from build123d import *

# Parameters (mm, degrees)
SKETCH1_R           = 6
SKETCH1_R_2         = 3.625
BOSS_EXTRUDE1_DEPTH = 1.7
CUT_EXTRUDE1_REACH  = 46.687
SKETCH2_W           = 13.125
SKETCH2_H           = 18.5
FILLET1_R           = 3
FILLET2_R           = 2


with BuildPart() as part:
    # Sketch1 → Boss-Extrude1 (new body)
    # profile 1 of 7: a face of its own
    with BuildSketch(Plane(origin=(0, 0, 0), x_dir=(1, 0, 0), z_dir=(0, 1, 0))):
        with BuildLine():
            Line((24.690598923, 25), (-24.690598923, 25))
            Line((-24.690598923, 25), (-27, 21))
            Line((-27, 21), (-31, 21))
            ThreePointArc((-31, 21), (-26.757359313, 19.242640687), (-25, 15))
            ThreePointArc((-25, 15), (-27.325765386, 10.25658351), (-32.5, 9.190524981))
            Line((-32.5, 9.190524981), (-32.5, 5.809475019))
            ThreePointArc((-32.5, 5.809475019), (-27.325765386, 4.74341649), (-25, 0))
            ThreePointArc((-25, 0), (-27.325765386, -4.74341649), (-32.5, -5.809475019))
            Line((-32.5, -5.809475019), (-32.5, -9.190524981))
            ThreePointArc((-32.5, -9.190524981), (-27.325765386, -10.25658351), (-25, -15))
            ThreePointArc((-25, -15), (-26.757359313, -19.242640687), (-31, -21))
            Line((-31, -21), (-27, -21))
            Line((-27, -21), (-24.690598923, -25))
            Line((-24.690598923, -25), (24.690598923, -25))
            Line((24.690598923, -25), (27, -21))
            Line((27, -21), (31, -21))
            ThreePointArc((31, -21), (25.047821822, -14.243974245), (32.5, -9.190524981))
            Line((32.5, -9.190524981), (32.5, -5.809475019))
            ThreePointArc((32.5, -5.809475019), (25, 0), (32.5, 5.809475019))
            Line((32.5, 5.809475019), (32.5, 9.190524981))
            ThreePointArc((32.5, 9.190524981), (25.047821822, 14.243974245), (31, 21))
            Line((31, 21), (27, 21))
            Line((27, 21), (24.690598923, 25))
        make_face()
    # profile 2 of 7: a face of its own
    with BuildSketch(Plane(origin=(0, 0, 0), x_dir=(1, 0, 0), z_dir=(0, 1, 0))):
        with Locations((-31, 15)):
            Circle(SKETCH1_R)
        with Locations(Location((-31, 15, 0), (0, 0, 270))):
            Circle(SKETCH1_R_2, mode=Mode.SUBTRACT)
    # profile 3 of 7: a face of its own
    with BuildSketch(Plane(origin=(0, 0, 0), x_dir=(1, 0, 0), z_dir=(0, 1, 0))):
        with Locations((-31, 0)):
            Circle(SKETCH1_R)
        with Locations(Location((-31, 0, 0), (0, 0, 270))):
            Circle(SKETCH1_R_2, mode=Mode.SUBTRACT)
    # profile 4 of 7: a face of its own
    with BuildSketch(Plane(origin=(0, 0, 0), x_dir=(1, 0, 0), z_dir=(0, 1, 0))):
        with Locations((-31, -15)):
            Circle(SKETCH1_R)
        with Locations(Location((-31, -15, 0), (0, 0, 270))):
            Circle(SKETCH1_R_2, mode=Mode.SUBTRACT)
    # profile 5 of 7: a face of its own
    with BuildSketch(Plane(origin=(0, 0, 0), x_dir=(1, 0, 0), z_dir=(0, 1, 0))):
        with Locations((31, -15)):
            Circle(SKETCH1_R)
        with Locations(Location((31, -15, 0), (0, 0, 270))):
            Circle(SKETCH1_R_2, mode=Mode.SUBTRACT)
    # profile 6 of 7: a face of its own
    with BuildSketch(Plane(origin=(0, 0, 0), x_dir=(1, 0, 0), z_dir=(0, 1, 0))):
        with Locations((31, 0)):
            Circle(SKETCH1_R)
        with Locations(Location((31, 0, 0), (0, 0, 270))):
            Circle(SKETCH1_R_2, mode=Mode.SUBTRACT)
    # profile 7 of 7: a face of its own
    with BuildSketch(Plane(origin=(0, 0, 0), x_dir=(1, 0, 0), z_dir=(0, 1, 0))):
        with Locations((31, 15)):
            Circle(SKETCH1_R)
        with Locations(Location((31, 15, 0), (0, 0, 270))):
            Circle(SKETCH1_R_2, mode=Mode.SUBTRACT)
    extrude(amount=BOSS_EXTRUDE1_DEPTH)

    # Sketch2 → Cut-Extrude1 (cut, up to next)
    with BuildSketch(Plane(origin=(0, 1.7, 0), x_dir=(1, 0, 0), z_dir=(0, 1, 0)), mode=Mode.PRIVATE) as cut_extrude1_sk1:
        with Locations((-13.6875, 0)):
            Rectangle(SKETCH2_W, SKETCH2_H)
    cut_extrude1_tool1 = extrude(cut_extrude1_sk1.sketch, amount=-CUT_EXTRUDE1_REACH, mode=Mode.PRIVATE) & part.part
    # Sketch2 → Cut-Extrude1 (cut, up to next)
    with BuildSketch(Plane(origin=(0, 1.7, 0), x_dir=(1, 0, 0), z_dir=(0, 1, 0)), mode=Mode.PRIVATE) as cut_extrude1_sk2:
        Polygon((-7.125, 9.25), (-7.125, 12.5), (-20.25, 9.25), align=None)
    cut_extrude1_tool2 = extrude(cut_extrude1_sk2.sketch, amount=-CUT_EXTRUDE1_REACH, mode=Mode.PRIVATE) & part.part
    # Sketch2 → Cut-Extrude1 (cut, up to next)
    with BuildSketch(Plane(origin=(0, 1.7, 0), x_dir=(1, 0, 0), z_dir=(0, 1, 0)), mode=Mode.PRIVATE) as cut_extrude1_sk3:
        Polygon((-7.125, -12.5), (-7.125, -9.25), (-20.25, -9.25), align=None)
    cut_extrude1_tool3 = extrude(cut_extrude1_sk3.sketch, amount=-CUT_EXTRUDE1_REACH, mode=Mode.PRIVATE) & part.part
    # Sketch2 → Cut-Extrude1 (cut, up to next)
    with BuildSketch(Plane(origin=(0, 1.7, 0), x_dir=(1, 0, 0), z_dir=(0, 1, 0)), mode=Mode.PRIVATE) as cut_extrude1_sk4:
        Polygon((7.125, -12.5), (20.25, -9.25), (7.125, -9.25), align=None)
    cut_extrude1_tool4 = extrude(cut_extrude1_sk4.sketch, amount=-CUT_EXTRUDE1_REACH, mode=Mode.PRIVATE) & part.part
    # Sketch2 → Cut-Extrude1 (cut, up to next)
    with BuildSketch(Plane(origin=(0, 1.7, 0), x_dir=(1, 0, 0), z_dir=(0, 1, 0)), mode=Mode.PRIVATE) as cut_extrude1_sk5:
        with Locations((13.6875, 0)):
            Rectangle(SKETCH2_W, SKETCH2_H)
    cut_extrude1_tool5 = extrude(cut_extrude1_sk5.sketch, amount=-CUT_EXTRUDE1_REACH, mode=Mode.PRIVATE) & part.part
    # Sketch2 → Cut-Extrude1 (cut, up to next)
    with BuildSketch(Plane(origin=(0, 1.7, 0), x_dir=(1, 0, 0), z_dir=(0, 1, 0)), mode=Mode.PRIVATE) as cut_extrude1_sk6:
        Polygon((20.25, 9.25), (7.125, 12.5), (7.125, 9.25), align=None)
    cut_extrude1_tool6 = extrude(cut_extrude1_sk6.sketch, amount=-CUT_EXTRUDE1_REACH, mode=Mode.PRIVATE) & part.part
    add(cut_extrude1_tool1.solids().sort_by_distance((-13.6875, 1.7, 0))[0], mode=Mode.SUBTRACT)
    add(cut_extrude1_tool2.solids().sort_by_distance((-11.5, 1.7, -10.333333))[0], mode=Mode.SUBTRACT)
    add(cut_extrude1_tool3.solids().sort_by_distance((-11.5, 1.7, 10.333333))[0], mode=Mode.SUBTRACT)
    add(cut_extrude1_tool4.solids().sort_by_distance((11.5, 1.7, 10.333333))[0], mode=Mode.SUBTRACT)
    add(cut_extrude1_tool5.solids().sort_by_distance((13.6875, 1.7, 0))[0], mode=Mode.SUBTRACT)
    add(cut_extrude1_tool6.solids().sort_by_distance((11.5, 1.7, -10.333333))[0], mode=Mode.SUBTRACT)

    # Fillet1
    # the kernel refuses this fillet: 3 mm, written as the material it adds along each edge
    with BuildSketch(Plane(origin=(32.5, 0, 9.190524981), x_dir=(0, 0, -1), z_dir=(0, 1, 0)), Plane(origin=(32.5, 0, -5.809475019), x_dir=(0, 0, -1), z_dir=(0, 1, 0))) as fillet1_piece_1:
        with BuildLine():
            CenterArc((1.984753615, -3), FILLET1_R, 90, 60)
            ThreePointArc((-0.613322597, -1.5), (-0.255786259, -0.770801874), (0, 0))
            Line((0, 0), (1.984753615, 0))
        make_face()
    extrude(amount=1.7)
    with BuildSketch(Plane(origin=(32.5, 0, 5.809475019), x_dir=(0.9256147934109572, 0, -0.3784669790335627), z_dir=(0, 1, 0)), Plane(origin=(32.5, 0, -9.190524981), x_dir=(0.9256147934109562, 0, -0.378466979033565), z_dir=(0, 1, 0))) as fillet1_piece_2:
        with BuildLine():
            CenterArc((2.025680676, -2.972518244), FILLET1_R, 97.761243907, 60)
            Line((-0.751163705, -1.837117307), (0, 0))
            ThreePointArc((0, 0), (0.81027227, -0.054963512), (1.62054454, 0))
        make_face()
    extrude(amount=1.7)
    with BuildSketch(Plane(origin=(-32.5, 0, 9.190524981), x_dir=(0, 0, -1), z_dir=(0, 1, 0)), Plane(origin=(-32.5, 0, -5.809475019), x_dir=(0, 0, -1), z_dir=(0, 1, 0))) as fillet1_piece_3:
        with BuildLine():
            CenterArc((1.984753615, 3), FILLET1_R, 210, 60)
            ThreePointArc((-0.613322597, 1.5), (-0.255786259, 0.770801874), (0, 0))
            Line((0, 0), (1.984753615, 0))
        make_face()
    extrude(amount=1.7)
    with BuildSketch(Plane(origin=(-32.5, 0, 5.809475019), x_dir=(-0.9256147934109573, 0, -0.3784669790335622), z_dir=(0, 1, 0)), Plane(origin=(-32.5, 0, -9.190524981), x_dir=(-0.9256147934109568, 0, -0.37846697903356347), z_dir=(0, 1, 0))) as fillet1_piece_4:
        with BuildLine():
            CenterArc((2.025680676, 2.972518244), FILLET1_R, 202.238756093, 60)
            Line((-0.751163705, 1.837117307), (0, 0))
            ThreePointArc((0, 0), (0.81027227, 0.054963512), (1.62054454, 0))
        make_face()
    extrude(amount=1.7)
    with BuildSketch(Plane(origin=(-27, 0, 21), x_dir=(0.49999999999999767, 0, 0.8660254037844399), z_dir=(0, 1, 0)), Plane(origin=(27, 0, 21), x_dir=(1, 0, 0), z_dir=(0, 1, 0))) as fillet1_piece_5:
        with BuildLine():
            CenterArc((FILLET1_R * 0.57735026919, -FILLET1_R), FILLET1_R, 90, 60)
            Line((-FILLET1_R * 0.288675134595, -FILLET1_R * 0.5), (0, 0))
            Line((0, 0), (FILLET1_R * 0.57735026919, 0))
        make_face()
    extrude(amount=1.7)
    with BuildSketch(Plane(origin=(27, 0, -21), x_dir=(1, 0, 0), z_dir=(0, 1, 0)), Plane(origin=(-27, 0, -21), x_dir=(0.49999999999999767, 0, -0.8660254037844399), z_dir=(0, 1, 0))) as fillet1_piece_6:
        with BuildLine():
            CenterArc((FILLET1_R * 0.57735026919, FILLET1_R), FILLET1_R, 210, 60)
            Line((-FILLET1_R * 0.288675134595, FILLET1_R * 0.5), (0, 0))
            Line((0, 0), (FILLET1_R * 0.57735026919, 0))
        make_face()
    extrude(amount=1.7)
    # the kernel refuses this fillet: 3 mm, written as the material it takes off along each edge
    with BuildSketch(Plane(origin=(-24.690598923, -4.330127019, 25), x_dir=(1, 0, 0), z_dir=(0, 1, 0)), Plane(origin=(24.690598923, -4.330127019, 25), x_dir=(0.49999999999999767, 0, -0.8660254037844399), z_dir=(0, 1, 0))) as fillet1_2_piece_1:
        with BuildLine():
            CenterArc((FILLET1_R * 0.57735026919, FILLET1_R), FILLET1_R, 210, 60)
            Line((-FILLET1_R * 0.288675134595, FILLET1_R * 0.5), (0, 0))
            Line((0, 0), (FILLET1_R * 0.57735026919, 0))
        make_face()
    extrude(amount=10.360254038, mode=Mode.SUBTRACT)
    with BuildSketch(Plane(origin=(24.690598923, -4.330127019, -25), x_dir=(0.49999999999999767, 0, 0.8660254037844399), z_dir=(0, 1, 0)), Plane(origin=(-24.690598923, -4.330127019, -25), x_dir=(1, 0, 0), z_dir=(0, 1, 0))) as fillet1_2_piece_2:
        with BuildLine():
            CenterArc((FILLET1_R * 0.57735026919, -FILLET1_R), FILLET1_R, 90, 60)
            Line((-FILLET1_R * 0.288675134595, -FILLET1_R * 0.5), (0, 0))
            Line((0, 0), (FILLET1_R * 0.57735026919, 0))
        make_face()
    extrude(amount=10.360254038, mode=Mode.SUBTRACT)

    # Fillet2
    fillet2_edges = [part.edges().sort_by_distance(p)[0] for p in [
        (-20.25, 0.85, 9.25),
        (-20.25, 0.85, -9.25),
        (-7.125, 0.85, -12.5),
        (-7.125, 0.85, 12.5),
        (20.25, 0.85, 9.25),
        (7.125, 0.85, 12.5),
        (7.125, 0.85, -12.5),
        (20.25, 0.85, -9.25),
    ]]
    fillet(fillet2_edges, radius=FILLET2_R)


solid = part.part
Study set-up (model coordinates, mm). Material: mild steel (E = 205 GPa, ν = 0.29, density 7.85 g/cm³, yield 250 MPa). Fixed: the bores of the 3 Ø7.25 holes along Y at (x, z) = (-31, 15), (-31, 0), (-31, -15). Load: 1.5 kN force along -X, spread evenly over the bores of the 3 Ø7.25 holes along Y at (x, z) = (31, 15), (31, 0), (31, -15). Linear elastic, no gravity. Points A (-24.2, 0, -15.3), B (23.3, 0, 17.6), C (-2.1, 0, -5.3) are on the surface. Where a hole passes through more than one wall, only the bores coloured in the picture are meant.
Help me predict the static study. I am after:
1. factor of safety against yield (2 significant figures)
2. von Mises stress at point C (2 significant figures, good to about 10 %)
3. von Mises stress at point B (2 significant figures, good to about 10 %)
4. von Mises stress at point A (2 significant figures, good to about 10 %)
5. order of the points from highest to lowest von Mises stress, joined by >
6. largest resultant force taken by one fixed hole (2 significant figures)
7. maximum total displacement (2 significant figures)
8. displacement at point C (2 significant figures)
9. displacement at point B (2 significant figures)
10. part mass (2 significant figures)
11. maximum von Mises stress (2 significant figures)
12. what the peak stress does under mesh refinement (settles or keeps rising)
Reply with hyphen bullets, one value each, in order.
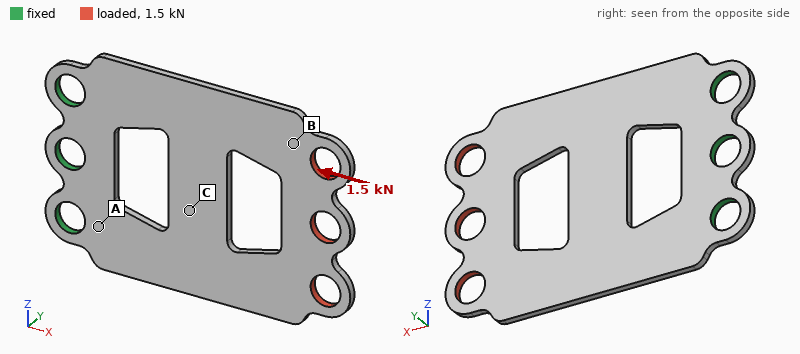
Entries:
- 2.3
- 6.7 MPa
- 23 MPa
- 41 MPa
- A > B > C
- 700 N
- 14 µm
- 4.5 µm
- 8.2 µm
- 34 g
- 110 MPa
- settles
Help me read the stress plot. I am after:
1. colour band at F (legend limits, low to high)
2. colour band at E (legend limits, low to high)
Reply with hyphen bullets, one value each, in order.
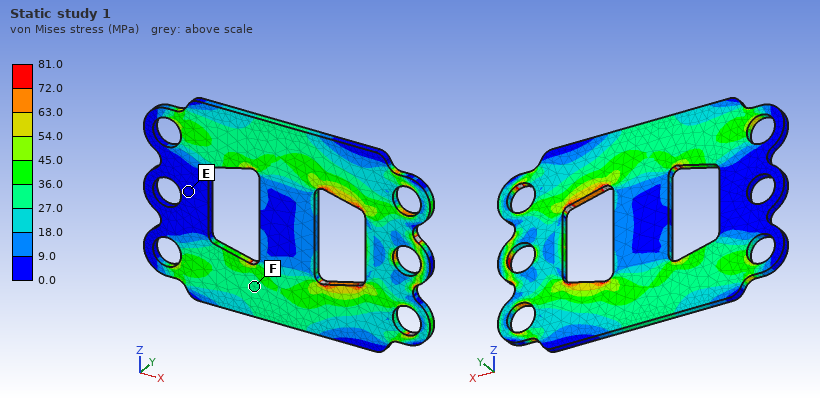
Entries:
- 27.0 to 36.0 MPa
- 0.0 to 9.0 MPa
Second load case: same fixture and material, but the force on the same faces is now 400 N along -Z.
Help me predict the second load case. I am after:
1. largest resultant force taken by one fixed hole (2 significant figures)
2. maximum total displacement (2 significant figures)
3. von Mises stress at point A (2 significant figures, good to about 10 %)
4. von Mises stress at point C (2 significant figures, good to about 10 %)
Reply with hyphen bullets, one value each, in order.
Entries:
- 670 N
- 35 µm
- 36 MPa
- 26 MPa
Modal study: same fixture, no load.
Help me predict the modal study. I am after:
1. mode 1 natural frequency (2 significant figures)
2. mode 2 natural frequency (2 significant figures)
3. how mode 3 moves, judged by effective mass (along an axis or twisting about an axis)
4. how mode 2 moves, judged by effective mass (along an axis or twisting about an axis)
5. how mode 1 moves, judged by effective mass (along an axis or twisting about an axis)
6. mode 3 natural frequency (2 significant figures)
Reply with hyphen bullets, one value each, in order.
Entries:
- 330 Hz
- 1000 Hz
- along Y
- twisting about X
- along Y
- 1900 Hz
